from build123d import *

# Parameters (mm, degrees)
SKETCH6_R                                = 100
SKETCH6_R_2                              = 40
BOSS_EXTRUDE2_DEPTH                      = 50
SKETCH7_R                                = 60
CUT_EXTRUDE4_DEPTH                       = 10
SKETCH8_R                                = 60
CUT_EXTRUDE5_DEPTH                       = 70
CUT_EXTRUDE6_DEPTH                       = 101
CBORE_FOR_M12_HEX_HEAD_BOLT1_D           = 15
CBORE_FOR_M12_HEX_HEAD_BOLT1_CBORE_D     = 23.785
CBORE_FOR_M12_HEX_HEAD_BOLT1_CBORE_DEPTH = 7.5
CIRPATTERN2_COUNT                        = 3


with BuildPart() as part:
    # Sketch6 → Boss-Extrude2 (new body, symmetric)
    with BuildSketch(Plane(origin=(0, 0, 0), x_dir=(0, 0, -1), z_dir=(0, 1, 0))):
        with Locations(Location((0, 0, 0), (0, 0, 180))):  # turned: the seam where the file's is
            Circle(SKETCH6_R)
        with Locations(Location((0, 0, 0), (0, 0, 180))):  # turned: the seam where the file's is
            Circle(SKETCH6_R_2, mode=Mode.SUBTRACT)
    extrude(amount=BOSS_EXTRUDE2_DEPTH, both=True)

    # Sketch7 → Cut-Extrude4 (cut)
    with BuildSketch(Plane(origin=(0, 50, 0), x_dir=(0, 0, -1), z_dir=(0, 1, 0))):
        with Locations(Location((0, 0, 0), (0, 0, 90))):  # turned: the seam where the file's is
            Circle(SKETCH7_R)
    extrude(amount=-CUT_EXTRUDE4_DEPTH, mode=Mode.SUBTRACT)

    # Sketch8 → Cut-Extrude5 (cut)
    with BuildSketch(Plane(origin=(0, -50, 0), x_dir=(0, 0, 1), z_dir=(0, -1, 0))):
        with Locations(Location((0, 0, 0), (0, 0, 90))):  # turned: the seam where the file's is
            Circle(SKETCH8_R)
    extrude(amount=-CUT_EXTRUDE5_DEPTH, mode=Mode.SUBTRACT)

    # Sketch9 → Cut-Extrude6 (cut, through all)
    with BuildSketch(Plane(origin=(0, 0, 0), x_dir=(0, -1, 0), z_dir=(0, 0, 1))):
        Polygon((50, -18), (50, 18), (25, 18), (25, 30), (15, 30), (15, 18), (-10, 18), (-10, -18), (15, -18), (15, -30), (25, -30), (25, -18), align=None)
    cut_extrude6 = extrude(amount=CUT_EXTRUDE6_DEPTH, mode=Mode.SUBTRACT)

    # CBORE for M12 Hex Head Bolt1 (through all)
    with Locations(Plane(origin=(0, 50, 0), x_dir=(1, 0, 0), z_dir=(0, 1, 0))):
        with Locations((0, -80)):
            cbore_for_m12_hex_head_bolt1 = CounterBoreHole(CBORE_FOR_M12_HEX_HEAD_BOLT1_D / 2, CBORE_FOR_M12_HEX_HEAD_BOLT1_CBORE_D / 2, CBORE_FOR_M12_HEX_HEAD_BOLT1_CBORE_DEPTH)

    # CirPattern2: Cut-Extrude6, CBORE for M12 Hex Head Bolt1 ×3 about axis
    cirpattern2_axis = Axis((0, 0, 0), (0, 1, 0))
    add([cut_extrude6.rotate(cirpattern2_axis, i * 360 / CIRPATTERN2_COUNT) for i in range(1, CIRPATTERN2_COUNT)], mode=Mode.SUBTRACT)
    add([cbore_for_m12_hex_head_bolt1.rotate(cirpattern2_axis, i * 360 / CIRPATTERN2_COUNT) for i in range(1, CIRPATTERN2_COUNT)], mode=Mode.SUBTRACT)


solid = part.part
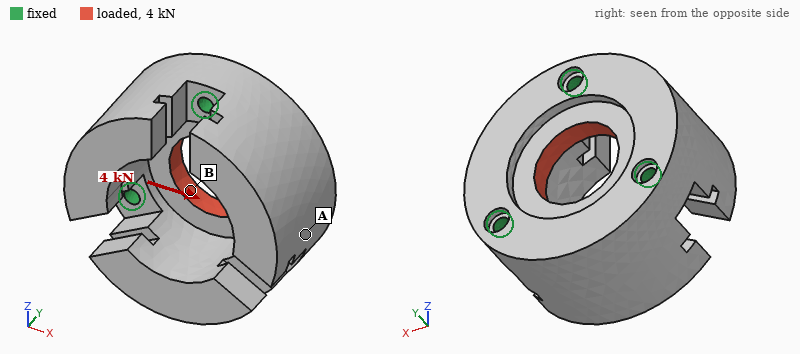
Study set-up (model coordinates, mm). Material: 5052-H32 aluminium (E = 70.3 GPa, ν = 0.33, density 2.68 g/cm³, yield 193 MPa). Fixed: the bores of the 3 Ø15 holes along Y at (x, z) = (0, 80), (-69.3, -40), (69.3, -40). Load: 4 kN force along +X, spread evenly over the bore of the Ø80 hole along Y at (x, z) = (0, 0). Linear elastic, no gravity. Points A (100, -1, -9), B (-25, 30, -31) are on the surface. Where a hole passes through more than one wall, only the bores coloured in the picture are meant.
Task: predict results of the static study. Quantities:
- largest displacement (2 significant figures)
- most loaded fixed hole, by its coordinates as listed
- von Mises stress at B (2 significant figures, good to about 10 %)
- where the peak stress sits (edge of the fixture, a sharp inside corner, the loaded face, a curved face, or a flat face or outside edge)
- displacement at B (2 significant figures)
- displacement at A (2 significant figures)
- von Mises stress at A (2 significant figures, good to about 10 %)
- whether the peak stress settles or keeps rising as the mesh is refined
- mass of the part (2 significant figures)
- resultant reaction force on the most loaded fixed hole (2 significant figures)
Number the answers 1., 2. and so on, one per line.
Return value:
1. 1.1 µm
2. (0, 80)
3. 1.3 MPa
4. edge of the fixture
5. 0.60 µm
6. 0.31 µm
7. 0.25 MPa
8. keeps rising
9. 4.9 kg
10. 1.6 kN
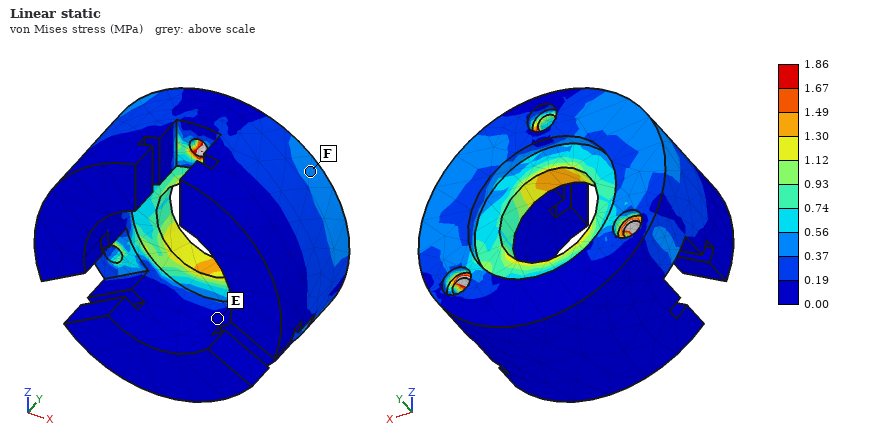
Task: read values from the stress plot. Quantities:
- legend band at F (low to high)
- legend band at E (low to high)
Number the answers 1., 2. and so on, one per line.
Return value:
1. 0.37 to 0.56 MPa
2. 0.00 to 0.19 MPa
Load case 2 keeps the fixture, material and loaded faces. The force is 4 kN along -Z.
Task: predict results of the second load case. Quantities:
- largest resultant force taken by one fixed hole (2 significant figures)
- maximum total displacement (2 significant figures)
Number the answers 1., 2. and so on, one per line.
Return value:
1. 1.5 kN
2. 1.2 µm
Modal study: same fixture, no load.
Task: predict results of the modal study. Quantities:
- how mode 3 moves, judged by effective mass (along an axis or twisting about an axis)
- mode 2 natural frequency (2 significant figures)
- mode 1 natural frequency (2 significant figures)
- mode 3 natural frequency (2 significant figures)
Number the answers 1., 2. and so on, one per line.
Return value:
1. along Y
2. 2100 Hz
3. 2100 Hz
4. 2200 Hz
